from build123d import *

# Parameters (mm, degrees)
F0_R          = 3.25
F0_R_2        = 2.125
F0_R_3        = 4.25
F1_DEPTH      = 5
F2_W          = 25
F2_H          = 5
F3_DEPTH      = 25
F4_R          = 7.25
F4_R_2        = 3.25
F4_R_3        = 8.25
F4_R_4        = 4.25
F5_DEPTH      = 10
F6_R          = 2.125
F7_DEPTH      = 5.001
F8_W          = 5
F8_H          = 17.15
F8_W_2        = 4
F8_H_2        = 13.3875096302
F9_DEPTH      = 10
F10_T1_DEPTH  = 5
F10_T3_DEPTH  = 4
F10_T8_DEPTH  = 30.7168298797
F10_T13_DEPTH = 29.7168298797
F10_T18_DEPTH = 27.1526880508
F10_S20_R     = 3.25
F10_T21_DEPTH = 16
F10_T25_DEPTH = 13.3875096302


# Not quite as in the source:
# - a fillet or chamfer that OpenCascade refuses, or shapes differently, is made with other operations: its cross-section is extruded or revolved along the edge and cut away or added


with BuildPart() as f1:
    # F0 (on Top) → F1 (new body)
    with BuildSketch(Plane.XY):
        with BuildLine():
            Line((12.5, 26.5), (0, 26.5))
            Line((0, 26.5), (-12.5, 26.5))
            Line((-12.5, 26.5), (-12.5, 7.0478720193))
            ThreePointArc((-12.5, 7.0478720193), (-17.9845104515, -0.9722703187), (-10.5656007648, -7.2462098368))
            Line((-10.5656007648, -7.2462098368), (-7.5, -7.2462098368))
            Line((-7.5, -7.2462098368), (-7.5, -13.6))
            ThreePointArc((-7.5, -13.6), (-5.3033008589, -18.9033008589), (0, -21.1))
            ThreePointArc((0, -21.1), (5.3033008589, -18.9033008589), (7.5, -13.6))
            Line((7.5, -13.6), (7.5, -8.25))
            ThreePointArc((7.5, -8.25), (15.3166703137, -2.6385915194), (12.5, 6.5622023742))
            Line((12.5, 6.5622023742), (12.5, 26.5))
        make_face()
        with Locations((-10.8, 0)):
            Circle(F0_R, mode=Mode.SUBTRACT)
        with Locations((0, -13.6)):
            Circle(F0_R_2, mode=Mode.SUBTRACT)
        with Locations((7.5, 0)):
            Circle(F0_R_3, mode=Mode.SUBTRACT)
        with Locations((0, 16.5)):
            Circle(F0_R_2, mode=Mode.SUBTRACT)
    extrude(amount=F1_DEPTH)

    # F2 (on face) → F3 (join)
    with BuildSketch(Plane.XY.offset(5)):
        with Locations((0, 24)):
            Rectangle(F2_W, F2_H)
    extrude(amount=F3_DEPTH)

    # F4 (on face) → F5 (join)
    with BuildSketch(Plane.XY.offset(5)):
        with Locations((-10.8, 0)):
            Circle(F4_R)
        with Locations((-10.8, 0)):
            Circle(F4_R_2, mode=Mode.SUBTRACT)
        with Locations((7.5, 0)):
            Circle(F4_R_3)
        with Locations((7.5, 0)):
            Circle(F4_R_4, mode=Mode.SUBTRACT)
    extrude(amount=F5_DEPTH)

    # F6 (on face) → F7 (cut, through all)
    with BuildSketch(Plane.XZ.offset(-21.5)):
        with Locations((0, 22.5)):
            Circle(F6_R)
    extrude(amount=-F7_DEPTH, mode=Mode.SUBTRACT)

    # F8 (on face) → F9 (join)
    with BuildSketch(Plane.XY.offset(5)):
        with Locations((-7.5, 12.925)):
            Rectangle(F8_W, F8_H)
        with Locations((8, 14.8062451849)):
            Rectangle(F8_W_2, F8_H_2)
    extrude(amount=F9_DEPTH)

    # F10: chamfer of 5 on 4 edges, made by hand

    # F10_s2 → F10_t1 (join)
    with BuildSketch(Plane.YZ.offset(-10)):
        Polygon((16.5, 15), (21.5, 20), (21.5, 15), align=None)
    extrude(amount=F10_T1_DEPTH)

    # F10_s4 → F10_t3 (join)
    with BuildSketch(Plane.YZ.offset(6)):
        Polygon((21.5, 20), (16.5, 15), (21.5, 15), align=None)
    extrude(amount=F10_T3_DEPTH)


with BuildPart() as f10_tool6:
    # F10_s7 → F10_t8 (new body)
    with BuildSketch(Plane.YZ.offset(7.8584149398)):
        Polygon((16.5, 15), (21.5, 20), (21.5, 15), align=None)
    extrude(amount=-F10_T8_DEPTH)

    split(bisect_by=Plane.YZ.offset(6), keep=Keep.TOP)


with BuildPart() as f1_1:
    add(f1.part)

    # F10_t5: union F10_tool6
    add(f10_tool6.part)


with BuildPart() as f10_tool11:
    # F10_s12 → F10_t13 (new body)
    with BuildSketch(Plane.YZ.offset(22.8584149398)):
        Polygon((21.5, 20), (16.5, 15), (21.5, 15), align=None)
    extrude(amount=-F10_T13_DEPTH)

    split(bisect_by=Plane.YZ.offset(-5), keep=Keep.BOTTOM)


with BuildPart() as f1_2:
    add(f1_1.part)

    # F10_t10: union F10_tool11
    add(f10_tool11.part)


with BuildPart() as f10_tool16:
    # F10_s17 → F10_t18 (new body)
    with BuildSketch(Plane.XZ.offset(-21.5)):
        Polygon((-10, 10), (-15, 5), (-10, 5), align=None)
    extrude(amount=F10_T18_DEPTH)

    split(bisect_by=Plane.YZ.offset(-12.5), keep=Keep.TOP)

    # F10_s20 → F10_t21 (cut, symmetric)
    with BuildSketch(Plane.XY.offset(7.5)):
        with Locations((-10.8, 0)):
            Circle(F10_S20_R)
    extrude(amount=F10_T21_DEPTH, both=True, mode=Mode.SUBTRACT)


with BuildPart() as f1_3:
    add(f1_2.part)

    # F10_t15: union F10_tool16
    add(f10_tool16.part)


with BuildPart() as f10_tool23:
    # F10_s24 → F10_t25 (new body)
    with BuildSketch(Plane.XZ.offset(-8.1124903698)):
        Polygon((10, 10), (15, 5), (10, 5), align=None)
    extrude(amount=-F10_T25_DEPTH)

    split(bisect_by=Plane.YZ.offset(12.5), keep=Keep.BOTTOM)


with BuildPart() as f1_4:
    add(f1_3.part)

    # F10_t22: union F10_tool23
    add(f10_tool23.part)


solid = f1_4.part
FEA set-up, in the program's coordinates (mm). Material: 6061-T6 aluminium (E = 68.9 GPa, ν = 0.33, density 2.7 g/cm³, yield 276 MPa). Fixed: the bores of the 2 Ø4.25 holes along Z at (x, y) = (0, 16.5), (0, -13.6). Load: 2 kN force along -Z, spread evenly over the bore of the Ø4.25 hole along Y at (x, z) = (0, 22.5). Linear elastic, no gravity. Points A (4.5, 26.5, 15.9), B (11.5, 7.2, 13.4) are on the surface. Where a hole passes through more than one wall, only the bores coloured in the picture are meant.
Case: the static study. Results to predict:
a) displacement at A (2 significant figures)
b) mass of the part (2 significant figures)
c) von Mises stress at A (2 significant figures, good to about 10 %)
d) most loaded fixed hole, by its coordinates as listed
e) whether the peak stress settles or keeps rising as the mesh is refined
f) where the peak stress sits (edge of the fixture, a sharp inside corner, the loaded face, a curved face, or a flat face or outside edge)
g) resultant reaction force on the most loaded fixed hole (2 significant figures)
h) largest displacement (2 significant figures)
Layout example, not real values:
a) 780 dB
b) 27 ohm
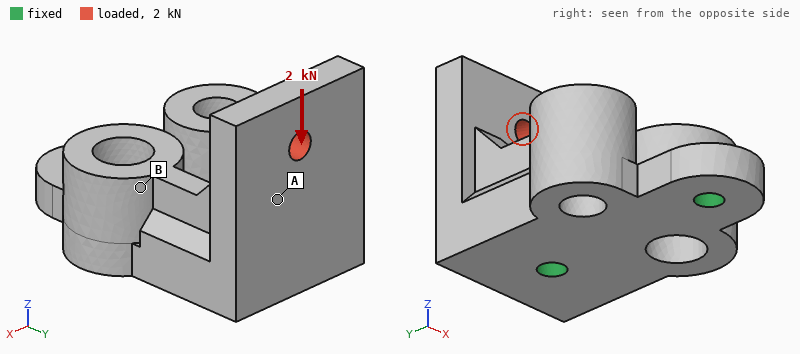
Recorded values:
a) 22 µm
b) 34 g
c) 26 MPa
d) (0, 16.5)
e) keeps rising
f) edge of the fixture
g) 2.4 kN
h) 35 µm
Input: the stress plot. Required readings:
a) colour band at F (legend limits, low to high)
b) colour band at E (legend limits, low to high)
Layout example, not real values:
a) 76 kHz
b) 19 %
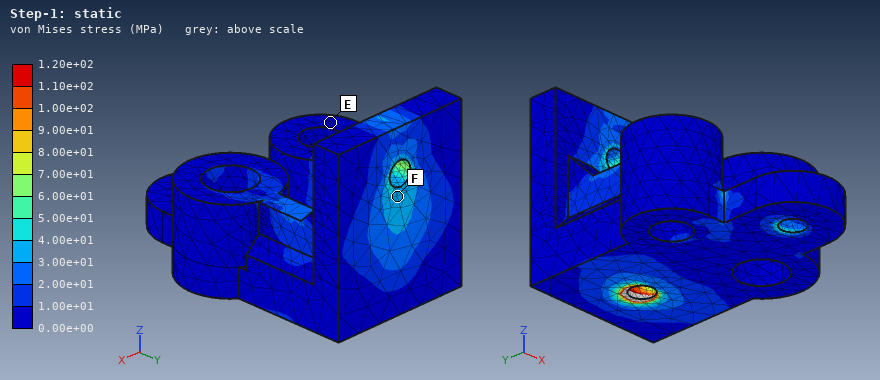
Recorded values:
a) 3.00e+01 to 4.00e+01 MPa
b) 0.00e+00 to 1.00e+01 MPa
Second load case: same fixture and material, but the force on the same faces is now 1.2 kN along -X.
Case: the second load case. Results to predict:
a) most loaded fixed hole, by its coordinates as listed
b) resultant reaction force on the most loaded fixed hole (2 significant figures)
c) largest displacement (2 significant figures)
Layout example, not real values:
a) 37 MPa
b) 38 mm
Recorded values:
a) (0, 16.5)
b) 1.4 kN
c) 0.13 mm
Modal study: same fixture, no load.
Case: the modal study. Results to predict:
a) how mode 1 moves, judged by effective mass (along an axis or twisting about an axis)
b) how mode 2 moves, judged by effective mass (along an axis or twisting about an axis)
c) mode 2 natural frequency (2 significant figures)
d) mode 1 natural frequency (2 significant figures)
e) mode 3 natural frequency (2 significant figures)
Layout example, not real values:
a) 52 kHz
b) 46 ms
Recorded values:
a) along X
b) along Y
c) 9400 Hz
d) 5800 Hz
e) 13 kHz
